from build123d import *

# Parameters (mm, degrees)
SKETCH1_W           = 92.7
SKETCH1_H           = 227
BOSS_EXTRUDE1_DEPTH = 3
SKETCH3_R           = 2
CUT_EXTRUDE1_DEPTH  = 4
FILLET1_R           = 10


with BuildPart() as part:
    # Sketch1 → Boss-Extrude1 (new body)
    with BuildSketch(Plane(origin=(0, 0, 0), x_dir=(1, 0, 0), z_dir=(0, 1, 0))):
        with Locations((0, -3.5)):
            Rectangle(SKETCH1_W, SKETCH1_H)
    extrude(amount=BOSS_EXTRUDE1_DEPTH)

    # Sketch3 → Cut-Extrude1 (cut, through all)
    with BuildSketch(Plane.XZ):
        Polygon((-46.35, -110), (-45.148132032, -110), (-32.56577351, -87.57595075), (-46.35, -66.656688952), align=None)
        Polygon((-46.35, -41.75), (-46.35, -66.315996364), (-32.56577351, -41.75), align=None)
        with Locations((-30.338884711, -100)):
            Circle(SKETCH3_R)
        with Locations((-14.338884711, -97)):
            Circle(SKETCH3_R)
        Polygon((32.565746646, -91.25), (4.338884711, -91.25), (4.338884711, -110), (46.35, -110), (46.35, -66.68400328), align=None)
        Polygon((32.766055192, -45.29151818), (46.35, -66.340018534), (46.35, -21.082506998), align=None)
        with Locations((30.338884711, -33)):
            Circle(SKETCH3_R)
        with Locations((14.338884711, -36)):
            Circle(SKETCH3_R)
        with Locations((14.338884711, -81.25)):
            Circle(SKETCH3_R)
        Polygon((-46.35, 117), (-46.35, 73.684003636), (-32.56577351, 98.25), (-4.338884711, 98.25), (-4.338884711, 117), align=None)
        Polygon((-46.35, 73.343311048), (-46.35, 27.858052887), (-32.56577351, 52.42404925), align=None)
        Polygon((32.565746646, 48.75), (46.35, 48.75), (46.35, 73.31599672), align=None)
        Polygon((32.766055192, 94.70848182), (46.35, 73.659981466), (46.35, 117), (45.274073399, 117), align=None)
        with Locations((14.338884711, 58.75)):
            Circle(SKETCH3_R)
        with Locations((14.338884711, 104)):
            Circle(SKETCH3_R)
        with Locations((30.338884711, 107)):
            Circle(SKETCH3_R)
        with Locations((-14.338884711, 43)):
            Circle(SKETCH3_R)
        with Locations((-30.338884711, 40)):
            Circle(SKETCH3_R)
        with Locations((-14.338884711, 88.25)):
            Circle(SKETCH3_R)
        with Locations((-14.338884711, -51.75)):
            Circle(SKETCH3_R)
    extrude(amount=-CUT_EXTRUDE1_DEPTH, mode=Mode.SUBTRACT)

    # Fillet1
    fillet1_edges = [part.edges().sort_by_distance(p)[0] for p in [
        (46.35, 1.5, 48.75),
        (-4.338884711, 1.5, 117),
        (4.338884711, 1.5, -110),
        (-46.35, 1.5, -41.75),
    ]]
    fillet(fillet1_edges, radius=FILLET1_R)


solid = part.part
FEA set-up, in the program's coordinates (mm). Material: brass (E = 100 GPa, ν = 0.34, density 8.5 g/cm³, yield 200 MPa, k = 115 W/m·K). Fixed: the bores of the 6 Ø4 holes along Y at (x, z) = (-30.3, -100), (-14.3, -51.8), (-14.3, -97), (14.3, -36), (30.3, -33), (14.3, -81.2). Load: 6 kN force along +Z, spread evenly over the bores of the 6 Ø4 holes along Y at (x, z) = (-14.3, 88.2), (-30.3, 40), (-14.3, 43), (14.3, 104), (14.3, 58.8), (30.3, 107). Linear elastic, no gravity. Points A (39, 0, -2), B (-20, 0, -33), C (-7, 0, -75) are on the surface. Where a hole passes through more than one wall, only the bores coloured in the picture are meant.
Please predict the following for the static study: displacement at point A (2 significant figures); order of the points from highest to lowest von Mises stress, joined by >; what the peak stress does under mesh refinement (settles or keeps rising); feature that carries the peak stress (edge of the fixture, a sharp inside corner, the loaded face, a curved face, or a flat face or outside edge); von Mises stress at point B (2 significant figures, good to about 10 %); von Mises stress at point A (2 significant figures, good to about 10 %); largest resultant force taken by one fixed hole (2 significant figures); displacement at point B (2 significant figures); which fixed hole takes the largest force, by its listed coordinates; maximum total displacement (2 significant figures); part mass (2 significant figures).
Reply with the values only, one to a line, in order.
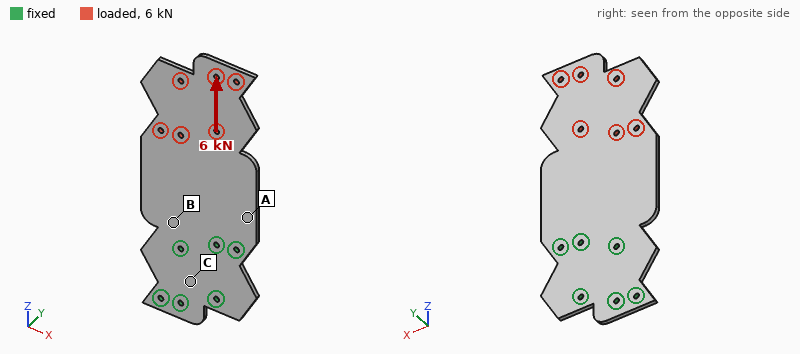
6.9 µm
B > A > C
keeps rising
edge of the fixture
29 MPa
17 MPa
2.2 kN
9.2 µm
(-14.3, -51.8)
41 µm
440 g
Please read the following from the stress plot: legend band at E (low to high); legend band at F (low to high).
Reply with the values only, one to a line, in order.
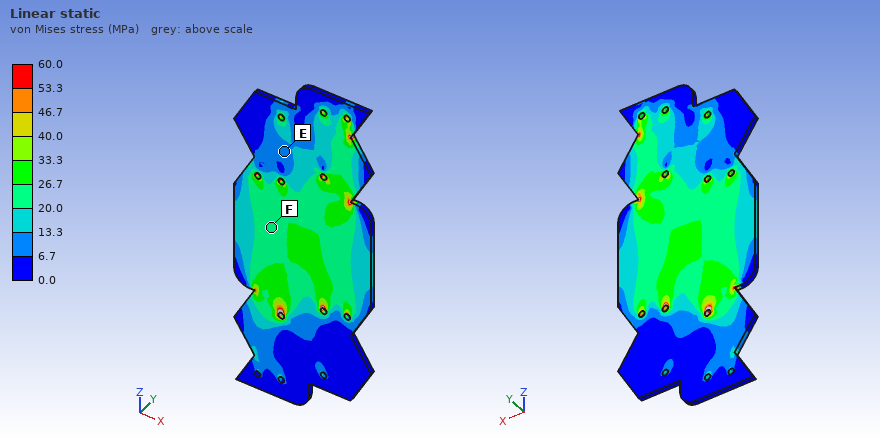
6.7 to 13.3 MPa
20.0 to 26.7 MPa
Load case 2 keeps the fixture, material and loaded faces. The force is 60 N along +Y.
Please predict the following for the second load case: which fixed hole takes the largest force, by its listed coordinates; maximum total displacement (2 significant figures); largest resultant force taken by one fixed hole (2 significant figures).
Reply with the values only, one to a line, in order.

(14.3, -36)
2.3 mm
120 N
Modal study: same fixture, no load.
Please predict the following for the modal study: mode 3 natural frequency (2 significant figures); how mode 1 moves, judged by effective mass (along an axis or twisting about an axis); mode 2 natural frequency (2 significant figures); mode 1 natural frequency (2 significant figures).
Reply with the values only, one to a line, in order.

470 Hz
along Y
280 Hz
81 Hz
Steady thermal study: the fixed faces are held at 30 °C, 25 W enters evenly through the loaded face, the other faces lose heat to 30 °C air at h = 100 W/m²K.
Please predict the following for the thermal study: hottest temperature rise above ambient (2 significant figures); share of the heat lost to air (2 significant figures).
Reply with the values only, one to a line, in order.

25 K
92 %
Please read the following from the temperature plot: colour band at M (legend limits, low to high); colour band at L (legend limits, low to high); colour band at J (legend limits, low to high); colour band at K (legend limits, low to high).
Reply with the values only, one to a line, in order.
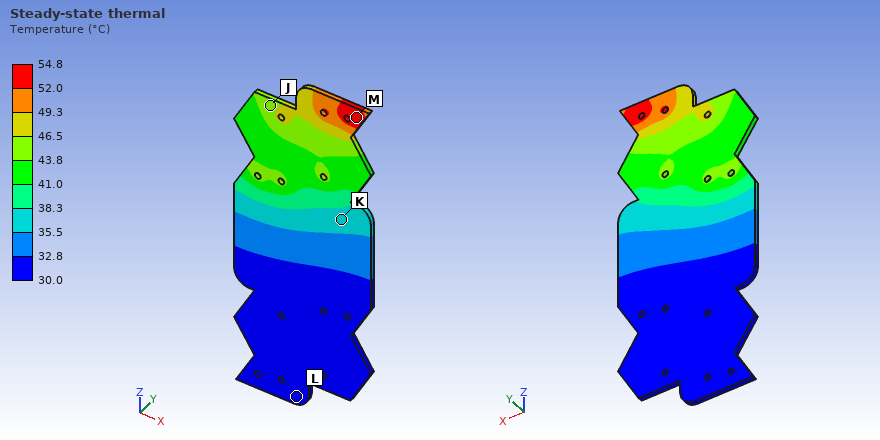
52.0 to 54.8 °C
30.0 to 32.8 °C
43.8 to 46.5 °C
35.5 to 38.3 °C
